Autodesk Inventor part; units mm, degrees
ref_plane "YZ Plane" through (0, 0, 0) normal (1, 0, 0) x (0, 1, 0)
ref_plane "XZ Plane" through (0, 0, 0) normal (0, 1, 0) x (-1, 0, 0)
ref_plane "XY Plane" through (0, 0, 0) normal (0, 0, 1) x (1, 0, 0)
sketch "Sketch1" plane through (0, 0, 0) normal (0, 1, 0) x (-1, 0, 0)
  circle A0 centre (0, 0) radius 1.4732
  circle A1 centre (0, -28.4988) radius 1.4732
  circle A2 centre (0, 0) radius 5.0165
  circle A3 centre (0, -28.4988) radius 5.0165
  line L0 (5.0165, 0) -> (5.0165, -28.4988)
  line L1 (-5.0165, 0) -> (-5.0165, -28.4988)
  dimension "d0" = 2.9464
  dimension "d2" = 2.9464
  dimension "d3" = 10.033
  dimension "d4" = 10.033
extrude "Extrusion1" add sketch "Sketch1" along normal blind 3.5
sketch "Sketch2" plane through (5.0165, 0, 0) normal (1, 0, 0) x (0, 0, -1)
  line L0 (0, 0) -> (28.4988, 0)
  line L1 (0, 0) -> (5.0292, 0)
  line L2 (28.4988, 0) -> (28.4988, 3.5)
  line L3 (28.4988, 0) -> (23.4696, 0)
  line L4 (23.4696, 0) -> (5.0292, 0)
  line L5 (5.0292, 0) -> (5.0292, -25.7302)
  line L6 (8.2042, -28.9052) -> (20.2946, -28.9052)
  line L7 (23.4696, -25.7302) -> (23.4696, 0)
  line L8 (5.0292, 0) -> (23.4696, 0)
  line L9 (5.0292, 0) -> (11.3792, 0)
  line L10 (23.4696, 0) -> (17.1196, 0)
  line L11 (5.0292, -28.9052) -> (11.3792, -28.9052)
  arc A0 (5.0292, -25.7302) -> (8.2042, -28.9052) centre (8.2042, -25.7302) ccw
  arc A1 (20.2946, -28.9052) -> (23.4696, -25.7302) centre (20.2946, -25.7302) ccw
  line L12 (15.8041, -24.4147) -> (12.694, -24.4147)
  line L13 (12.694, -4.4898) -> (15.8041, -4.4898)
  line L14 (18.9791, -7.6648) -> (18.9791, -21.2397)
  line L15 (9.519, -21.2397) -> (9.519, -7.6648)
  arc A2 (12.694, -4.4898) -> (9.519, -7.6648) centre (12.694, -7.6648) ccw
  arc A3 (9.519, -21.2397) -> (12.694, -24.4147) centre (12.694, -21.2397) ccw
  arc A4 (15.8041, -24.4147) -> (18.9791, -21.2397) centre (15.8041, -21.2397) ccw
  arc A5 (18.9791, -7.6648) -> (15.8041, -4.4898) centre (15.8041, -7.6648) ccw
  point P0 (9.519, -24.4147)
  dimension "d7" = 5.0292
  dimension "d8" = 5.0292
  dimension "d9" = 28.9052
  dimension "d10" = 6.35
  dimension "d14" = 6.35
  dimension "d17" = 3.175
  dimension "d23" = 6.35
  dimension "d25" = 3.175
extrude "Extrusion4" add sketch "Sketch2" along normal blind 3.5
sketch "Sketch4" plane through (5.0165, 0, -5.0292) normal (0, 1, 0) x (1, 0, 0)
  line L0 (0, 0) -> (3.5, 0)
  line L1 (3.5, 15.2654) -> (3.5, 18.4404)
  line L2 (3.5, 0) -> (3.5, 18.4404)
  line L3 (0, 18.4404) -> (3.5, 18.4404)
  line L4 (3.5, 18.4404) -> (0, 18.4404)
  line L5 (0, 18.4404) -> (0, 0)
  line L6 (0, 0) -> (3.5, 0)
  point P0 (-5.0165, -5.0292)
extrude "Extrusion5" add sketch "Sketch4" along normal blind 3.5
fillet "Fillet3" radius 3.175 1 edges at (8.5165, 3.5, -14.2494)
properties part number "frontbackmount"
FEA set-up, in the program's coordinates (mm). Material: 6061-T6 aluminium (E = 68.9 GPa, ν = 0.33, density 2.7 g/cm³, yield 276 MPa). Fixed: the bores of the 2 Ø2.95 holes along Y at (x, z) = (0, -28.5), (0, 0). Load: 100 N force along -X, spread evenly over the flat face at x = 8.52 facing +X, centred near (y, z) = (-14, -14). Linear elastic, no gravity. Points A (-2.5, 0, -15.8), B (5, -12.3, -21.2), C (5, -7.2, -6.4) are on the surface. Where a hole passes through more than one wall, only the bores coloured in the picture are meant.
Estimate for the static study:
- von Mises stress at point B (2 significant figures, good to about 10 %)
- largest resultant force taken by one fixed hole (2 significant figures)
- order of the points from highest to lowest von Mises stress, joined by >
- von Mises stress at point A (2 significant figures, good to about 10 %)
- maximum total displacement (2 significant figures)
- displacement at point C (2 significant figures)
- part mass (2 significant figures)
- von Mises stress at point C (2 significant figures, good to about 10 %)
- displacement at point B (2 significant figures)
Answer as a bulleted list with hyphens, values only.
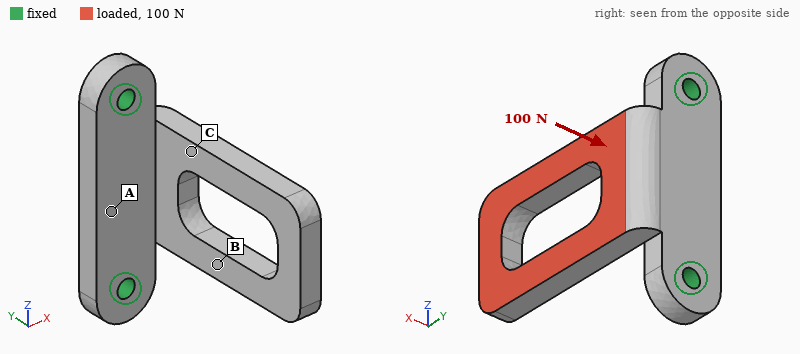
- 28 MPa
- 53 N
- C > B > A
- 9.1 MPa
- 0.22 mm
- 0.041 mm
- 7.1 g
- 40 MPa
- 0.076 mm
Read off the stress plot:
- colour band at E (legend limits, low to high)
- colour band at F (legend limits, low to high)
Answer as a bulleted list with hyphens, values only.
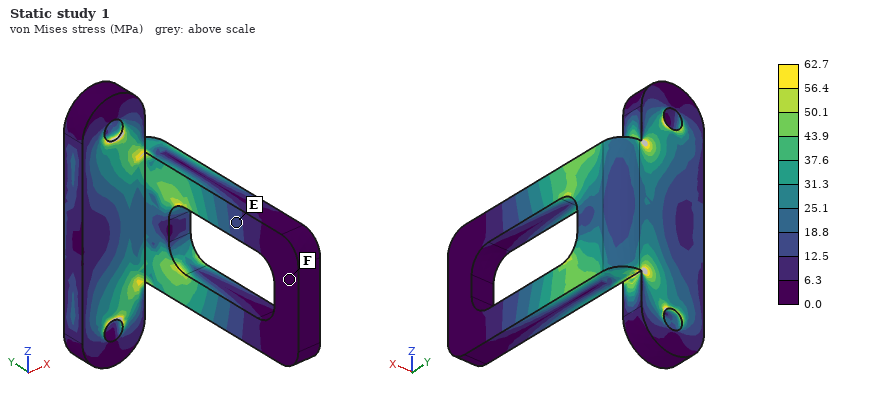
- 12.5 to 18.8 MPa
- 0.0 to 6.3 MPa
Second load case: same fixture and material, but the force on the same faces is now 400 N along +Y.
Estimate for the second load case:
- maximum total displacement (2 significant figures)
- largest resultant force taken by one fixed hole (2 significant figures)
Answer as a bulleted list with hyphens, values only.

- 0.23 mm
- 200 N
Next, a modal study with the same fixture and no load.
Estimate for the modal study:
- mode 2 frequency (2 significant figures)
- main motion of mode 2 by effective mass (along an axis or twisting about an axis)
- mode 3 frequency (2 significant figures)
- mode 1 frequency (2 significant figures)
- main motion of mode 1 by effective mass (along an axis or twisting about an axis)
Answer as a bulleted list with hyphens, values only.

- 5400 Hz
- along Z
- 7600 Hz
- 2200 Hz
- along X
